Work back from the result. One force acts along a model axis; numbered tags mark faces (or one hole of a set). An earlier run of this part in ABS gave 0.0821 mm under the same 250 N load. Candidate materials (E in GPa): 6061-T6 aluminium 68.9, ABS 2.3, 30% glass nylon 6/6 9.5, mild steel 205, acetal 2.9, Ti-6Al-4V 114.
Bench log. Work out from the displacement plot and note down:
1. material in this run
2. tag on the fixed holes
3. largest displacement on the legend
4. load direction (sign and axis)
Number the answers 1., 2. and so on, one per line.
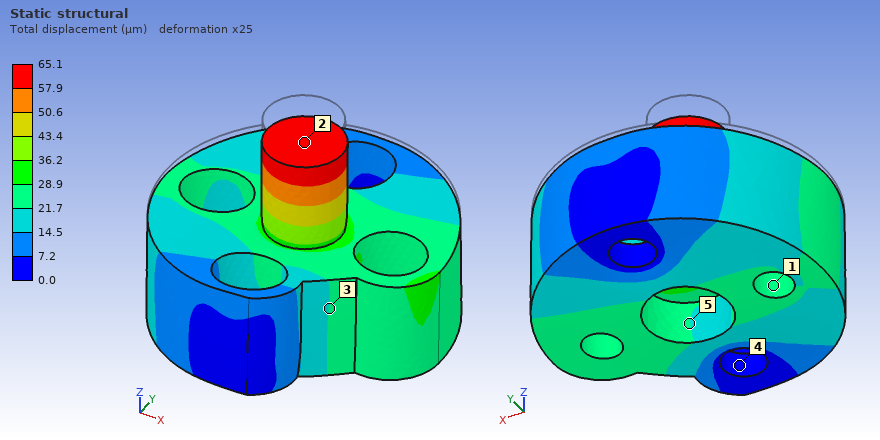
1. acetal
2. 4
3. 65.1 µm
4. -Z
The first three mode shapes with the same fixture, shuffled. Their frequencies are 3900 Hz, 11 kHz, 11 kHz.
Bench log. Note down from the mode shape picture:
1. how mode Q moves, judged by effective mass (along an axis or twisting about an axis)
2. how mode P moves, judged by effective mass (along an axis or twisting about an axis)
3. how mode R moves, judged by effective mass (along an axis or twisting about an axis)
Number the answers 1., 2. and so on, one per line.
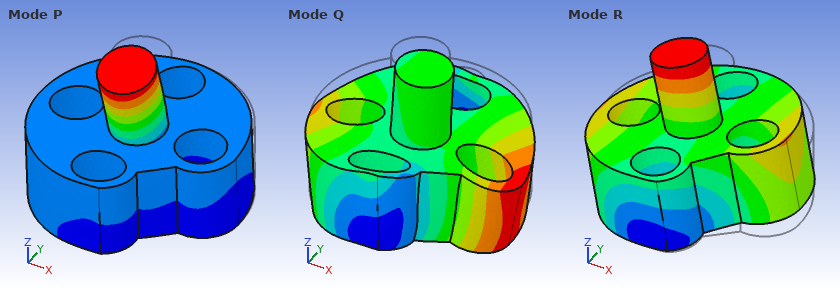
1. along Z
2. along Y
3. along X
